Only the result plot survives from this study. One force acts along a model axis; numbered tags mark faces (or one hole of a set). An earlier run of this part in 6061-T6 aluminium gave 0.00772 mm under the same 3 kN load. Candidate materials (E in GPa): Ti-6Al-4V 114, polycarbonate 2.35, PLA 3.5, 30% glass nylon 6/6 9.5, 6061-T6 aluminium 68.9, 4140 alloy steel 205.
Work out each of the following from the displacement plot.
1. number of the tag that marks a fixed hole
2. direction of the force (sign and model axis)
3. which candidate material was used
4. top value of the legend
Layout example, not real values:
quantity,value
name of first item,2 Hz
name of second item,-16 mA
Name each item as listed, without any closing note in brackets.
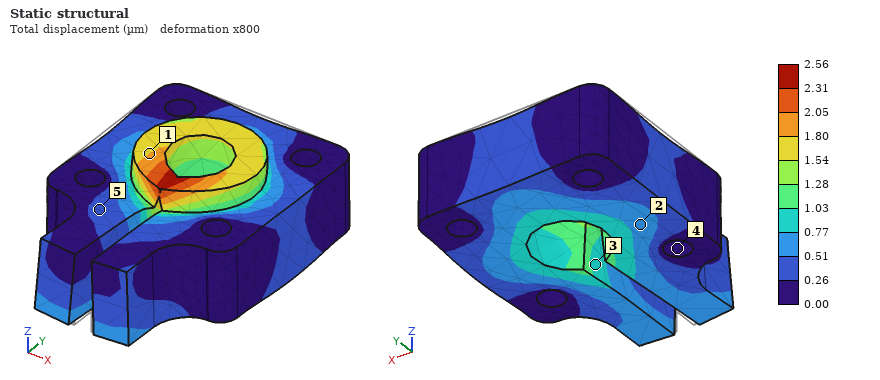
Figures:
quantity,value
number of the tag that marks a fixed hole,4
direction of the force,-Z
which candidate material was used,4140 alloy steel
top value of the legend,2.56 µm
